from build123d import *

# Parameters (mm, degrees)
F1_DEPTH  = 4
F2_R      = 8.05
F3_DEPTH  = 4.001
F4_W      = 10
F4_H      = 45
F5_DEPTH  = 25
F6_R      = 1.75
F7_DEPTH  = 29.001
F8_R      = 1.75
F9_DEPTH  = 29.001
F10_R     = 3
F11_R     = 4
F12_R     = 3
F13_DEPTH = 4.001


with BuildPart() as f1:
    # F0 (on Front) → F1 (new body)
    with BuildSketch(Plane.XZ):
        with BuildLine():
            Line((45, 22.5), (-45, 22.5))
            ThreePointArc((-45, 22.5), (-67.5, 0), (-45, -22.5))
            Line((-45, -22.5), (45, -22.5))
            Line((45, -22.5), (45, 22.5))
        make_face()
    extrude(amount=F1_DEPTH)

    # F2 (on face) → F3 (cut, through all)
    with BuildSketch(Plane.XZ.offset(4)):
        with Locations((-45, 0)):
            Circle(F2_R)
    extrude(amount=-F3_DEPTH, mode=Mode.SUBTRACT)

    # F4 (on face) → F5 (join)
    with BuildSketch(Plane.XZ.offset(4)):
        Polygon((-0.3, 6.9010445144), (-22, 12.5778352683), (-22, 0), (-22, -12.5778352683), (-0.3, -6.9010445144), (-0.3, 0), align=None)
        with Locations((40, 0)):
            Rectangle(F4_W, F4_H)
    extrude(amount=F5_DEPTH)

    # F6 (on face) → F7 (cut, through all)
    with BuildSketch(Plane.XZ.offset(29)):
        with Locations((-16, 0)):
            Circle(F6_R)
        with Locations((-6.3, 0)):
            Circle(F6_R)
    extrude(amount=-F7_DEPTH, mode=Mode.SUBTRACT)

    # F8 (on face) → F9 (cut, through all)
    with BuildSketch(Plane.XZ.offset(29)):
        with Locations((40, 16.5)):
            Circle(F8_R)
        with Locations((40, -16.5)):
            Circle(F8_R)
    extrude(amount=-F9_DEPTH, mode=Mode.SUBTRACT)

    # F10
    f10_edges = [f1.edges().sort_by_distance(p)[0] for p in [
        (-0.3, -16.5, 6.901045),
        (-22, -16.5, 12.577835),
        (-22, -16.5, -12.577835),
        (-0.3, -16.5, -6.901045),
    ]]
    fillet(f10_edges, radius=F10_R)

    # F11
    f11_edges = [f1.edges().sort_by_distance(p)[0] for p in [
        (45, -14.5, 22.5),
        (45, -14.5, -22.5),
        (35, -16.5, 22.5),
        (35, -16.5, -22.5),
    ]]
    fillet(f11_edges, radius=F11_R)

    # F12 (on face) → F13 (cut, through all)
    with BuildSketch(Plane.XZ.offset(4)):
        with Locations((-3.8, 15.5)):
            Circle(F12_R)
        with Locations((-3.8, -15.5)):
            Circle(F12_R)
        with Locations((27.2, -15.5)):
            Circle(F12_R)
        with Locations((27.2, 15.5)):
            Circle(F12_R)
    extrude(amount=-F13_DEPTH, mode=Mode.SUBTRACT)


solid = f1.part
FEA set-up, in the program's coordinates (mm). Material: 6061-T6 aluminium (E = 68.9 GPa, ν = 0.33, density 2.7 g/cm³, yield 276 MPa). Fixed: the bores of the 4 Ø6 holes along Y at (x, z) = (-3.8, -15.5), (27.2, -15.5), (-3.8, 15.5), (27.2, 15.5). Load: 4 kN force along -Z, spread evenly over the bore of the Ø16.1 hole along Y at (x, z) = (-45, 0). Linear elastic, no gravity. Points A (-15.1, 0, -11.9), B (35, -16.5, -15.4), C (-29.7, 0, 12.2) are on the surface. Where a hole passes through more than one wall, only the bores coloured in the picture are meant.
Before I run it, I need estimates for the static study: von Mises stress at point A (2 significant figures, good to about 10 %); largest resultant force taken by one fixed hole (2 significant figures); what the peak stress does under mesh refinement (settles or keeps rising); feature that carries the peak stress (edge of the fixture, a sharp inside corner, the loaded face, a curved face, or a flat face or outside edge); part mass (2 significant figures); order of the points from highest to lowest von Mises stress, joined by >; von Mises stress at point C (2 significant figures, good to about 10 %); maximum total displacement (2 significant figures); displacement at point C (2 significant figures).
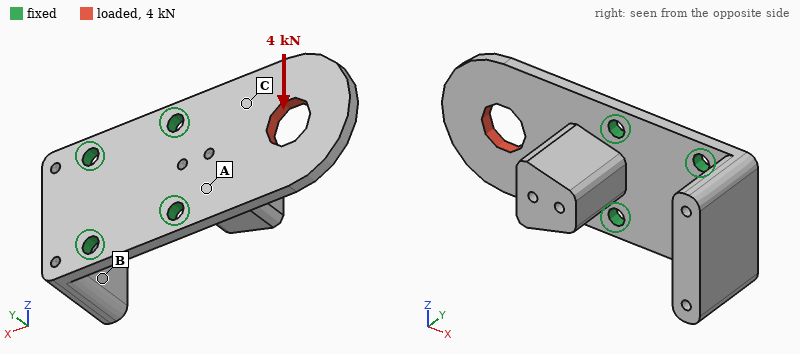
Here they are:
65 MPa
5.0 kN
keeps rising
edge of the fixture
100 g
A > C > B
41 MPa
0.13 mm
0.047 mm
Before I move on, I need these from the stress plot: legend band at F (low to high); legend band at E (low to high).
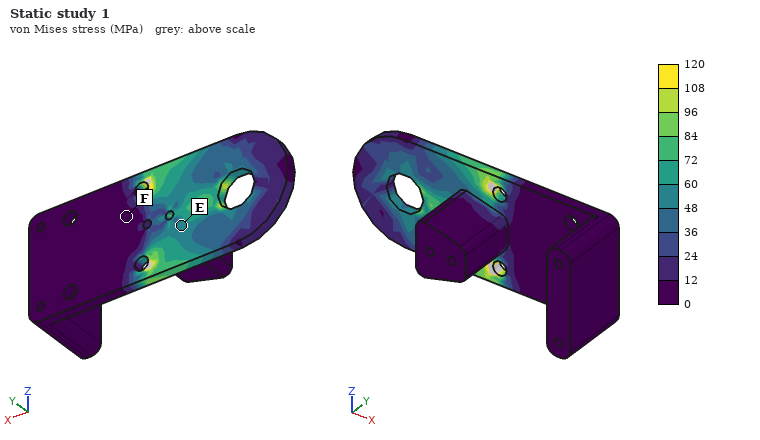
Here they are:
0 to 12 MPa
48 to 60 MPa
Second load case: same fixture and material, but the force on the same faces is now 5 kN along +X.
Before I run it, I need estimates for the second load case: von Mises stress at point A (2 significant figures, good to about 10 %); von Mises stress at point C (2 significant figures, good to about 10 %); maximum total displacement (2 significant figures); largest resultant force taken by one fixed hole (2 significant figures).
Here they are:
33 MPa
33 MPa
36 µm
2.2 kN
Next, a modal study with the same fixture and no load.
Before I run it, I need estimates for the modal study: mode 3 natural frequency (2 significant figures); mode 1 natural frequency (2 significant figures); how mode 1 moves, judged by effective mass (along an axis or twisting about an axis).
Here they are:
3700 Hz
1300 Hz
along Y
